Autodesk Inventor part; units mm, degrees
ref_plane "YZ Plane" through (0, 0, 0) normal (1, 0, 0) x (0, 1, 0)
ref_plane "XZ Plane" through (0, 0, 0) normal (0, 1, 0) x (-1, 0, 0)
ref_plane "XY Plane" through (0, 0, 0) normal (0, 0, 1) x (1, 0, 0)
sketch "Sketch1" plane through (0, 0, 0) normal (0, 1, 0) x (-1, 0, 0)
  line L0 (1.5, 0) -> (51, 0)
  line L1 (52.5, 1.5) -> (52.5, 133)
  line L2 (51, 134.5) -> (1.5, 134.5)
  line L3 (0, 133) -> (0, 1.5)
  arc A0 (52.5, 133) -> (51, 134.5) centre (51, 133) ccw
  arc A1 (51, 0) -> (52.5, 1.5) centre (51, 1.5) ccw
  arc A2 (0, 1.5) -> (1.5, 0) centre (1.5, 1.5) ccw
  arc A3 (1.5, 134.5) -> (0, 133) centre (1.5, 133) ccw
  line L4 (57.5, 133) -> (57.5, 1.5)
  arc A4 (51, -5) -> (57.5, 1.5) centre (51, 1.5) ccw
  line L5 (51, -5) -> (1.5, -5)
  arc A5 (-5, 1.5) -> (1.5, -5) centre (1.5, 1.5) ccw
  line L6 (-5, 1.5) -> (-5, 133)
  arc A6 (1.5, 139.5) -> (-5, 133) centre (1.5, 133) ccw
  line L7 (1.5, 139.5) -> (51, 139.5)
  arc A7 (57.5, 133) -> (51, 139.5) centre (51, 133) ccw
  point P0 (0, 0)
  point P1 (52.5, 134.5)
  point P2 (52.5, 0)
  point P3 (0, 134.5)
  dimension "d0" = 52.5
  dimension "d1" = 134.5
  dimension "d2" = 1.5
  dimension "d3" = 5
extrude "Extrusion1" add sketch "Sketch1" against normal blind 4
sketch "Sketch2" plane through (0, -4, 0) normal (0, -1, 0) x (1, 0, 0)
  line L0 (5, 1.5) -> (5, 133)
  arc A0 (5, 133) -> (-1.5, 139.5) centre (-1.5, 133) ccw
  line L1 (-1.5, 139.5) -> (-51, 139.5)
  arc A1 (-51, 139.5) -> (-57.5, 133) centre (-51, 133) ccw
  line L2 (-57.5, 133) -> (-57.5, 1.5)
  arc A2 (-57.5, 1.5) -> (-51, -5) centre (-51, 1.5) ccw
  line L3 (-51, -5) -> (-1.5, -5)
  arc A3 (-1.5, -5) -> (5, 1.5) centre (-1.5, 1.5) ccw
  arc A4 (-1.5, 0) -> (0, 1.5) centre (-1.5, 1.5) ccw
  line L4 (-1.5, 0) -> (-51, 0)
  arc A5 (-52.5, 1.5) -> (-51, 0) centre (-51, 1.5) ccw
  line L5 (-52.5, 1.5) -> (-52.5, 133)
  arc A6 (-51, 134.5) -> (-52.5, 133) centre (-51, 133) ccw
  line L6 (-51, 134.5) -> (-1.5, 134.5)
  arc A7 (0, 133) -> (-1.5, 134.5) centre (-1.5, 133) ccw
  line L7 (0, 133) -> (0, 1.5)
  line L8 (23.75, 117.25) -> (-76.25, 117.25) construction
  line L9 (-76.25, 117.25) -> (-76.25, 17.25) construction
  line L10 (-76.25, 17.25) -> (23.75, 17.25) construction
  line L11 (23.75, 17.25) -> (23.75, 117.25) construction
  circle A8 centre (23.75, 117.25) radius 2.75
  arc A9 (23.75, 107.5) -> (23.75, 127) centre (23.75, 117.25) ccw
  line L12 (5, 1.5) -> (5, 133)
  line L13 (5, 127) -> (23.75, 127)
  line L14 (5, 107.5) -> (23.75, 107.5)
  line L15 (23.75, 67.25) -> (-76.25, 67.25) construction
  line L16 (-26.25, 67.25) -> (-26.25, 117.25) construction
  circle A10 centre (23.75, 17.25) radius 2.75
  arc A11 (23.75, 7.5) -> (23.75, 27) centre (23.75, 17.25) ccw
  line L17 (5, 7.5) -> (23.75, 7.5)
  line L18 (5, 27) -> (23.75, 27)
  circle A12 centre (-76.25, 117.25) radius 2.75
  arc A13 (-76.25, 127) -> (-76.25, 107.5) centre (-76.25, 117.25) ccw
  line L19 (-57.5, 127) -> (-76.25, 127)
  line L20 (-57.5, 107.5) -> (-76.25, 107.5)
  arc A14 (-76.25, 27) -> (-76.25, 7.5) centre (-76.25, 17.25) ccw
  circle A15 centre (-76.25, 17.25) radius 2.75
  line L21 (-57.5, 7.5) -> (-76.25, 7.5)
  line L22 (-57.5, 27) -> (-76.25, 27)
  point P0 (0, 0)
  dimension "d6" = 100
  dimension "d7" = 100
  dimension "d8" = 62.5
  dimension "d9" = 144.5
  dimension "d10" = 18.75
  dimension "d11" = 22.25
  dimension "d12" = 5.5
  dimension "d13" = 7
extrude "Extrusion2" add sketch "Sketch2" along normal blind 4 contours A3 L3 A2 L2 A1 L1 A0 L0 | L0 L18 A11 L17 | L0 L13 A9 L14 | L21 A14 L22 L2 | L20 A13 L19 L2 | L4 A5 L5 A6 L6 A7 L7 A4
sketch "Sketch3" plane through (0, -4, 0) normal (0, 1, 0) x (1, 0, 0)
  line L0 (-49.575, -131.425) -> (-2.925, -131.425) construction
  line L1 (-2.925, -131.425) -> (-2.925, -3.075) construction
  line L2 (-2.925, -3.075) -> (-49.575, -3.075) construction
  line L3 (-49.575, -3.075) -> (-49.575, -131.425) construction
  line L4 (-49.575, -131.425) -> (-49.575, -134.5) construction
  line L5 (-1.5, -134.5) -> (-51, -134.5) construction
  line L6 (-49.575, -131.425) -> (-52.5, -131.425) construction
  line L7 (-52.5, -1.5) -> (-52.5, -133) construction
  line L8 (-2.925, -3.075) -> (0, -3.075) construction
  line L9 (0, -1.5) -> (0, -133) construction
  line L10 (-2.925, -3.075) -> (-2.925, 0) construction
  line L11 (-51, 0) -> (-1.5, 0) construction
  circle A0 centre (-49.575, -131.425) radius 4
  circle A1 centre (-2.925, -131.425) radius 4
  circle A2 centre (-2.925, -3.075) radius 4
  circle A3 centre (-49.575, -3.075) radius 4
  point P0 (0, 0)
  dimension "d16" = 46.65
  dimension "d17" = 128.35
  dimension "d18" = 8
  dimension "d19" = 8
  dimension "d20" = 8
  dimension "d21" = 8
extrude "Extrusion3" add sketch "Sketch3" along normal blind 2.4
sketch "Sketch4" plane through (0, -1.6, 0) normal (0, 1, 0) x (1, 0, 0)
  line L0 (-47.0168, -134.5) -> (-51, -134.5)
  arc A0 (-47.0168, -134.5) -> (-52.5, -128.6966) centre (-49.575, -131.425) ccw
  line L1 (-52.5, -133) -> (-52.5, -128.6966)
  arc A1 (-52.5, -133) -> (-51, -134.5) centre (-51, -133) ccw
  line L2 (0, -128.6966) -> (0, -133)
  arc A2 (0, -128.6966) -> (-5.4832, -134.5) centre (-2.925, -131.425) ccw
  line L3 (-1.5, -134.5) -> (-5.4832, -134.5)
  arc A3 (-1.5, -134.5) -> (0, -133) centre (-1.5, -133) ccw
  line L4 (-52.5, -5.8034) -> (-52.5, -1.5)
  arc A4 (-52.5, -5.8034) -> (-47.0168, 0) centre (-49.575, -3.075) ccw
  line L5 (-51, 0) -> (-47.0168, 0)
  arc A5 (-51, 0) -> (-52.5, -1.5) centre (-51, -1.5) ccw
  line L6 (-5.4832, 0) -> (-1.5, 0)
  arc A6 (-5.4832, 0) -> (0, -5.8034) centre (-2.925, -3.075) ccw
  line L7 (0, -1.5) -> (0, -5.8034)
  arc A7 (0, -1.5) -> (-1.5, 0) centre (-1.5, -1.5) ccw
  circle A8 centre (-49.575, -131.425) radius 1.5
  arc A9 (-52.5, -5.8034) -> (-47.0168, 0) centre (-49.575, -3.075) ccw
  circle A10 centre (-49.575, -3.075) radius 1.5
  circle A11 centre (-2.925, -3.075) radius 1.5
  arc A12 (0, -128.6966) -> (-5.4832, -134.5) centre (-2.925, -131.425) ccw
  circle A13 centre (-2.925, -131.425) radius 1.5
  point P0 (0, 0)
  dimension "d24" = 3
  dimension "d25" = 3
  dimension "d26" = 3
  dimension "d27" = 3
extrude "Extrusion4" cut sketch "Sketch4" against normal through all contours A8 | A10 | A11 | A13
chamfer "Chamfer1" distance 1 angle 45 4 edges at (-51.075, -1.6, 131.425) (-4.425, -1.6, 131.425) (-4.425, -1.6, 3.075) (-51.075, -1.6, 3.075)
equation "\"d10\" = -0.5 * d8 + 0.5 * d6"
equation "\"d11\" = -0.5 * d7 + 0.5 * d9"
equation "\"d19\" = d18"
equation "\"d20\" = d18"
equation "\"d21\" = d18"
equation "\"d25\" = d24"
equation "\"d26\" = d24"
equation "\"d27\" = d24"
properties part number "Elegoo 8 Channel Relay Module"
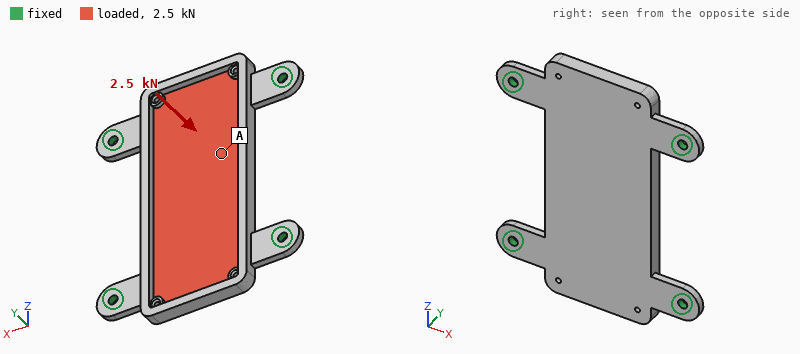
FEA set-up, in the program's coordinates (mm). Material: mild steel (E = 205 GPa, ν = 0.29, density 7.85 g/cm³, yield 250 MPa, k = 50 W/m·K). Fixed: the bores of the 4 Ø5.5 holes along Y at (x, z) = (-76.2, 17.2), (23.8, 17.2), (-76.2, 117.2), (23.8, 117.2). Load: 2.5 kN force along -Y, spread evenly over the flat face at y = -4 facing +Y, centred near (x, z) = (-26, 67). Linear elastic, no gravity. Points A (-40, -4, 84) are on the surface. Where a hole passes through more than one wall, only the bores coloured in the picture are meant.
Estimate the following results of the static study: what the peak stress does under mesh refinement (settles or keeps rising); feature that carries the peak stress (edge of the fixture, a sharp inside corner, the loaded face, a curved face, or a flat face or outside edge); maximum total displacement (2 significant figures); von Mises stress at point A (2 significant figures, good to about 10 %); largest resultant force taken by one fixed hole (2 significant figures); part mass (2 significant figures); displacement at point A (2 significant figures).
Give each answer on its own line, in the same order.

keeps rising
edge of the fixture
0.15 mm
39 MPa
650 N
410 g
0.13 mm
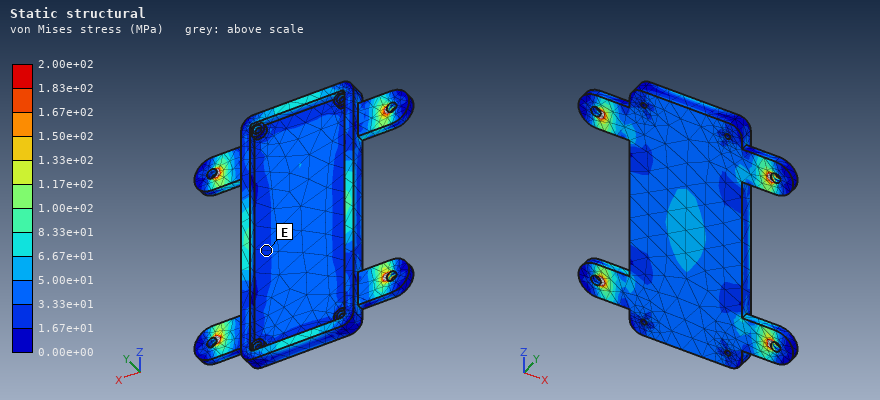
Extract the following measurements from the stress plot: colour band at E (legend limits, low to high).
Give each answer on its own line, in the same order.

1.67e+01 to 3.33e+01 MPa
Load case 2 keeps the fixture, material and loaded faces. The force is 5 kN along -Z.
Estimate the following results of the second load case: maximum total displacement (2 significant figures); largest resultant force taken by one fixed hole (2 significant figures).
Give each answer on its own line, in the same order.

23 µm
1.3 kN
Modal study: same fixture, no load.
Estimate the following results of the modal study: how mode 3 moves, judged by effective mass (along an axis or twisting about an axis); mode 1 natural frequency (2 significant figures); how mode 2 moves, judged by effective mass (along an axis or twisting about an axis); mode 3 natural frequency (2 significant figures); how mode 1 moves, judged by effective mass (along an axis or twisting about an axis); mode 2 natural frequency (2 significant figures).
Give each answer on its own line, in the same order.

along Y
1400 Hz
twisting about X
2200 Hz
along Y
2000 Hz
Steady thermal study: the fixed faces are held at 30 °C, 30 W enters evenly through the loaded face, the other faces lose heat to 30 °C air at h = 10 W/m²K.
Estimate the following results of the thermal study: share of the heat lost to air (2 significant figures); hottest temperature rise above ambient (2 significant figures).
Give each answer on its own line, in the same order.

23 %
51 K
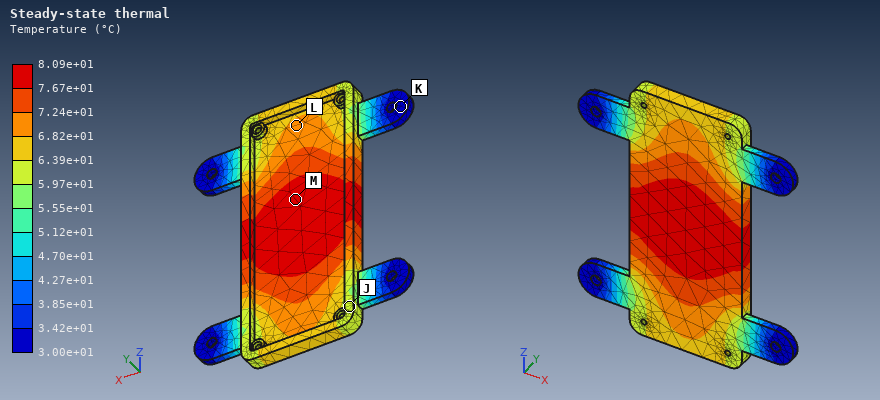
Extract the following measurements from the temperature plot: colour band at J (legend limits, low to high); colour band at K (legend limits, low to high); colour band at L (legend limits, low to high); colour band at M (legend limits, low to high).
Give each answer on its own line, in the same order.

5.97e+01 to 6.39e+01 °C
3.00e+01 to 3.42e+01 °C
6.82e+01 to 7.24e+01 °C
7.67e+01 to 8.09e+01 °C
